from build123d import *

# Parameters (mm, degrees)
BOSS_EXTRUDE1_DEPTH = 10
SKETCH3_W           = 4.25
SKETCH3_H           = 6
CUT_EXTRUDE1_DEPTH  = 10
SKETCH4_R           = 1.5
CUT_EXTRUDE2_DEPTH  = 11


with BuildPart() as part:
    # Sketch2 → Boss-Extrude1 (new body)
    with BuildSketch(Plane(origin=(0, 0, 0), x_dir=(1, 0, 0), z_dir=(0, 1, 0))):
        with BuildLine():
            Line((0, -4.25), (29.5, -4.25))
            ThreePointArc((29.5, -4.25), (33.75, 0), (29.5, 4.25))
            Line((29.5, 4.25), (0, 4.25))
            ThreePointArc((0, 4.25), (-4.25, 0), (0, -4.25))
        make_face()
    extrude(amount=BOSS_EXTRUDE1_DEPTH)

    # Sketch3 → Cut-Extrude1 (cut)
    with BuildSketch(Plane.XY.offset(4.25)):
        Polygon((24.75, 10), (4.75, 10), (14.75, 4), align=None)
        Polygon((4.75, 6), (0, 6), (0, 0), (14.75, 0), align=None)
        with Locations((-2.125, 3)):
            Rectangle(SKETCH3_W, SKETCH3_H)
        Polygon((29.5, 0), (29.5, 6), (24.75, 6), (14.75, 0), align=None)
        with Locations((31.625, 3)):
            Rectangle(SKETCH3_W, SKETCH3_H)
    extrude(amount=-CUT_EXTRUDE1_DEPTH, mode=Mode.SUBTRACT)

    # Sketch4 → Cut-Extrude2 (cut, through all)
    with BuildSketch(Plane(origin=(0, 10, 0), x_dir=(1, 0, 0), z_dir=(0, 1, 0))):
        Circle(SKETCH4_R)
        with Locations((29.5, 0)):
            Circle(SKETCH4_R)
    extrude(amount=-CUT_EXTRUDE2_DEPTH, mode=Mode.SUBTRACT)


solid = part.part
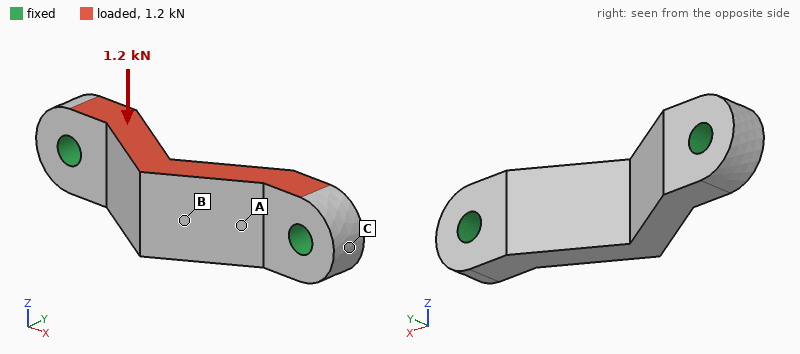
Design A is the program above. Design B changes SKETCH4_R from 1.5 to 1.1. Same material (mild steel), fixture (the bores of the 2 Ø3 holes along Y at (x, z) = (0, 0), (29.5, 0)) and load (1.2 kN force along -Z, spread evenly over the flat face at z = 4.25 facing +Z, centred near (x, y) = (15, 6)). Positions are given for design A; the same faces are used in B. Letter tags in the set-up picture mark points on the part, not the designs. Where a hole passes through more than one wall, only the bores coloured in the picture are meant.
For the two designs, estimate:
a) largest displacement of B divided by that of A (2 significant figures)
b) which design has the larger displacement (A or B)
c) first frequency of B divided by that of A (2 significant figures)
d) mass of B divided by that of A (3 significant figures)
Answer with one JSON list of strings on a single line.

["1.3", "B", "0.89", "1.02"]
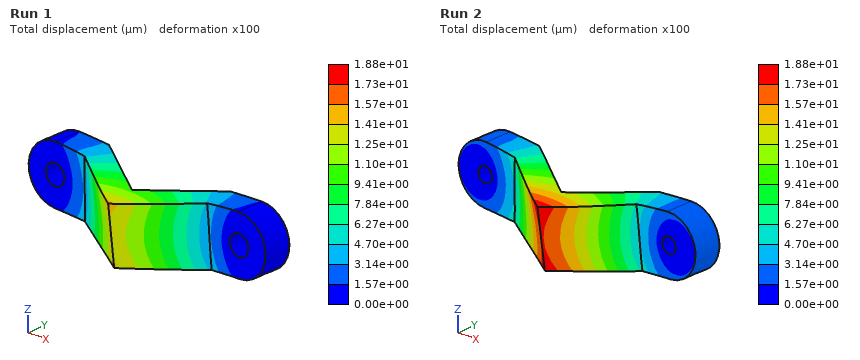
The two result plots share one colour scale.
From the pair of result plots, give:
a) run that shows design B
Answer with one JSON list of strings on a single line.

["Run 2"]
